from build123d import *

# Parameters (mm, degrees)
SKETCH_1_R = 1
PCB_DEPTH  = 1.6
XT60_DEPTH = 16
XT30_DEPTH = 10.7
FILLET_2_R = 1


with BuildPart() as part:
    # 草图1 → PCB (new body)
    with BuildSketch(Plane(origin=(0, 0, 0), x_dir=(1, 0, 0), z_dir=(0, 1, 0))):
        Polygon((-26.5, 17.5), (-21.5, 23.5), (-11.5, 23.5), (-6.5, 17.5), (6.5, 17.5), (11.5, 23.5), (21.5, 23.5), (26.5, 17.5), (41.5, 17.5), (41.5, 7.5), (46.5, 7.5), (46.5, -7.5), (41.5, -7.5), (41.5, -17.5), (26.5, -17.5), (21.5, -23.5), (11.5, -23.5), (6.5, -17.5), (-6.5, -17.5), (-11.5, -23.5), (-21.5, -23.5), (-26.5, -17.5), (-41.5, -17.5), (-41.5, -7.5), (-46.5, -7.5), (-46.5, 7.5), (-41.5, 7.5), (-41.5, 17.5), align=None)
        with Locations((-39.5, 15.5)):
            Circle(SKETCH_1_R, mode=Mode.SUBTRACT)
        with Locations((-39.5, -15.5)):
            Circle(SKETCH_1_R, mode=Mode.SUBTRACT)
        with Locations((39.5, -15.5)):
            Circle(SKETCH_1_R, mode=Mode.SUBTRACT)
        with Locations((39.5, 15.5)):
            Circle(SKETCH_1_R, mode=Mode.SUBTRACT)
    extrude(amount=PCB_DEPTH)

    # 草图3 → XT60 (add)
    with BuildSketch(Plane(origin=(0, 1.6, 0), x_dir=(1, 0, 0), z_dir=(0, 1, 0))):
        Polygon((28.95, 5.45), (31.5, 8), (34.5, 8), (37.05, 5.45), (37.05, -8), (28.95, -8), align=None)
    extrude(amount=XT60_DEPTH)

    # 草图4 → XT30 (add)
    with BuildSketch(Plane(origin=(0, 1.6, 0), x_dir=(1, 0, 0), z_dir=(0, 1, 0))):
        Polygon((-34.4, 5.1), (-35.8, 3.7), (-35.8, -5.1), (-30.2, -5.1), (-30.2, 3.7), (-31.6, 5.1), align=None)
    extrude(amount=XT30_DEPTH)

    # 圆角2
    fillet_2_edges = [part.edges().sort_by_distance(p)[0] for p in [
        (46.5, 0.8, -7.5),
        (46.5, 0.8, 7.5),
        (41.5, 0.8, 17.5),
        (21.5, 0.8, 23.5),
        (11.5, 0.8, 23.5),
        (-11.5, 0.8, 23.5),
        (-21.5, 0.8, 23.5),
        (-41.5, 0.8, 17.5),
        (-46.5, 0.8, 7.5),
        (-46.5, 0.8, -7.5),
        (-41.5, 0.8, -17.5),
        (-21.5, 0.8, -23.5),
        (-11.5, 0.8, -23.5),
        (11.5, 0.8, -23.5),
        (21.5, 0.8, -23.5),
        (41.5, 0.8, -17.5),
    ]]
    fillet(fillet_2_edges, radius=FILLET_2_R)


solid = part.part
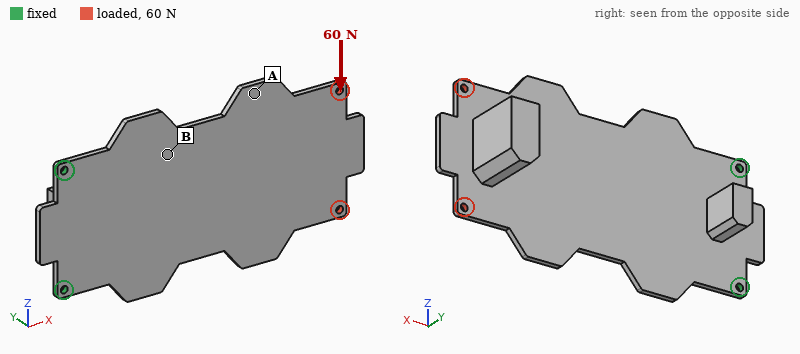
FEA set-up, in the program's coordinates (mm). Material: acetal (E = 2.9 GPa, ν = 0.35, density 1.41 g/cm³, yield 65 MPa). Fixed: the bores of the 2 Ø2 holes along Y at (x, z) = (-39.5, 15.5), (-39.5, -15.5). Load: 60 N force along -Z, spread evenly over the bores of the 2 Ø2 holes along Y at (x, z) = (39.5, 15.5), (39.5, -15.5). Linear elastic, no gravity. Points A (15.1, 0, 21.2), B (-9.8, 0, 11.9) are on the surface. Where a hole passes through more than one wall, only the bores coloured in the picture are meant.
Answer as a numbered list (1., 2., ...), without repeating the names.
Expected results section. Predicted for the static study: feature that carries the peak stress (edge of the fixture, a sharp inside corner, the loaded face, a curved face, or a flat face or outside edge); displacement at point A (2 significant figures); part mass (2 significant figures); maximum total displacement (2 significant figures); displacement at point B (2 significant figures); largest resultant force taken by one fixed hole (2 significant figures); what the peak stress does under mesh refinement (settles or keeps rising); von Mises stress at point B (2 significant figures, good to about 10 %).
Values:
1. edge of the fixture
2. 0.45 mm
3. 11 g
4. 0.75 mm
5. 0.18 mm
6. 160 N
7. keeps rising
8. 5.1 MPa
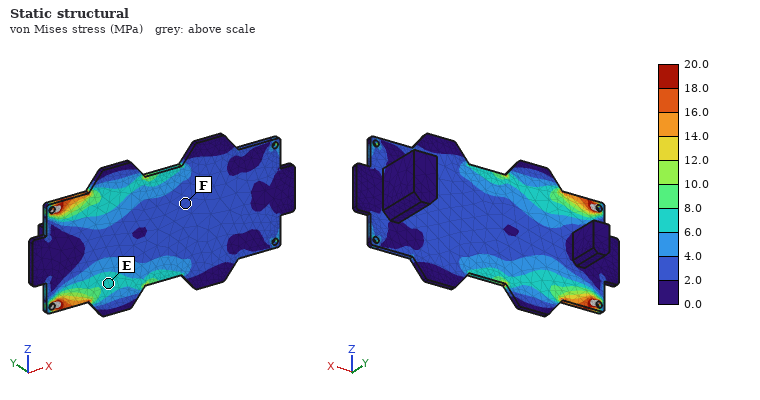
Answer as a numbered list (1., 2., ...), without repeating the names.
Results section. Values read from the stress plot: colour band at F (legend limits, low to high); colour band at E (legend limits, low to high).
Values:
1. 2.0 to 4.0 MPa
2. 6.0 to 8.0 MPa
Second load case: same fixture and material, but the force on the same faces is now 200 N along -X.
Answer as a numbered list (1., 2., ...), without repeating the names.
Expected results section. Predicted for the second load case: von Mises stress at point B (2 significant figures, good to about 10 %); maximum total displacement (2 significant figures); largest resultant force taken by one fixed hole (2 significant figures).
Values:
1. 3.4 MPa
2. 0.17 mm
3. 100 N
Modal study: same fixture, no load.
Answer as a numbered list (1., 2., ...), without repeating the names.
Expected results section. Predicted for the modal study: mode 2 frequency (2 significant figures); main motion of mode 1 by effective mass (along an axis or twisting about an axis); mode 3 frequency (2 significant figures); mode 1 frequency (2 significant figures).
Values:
1. 180 Hz
2. along Y
3. 250 Hz
4. 34 Hz
